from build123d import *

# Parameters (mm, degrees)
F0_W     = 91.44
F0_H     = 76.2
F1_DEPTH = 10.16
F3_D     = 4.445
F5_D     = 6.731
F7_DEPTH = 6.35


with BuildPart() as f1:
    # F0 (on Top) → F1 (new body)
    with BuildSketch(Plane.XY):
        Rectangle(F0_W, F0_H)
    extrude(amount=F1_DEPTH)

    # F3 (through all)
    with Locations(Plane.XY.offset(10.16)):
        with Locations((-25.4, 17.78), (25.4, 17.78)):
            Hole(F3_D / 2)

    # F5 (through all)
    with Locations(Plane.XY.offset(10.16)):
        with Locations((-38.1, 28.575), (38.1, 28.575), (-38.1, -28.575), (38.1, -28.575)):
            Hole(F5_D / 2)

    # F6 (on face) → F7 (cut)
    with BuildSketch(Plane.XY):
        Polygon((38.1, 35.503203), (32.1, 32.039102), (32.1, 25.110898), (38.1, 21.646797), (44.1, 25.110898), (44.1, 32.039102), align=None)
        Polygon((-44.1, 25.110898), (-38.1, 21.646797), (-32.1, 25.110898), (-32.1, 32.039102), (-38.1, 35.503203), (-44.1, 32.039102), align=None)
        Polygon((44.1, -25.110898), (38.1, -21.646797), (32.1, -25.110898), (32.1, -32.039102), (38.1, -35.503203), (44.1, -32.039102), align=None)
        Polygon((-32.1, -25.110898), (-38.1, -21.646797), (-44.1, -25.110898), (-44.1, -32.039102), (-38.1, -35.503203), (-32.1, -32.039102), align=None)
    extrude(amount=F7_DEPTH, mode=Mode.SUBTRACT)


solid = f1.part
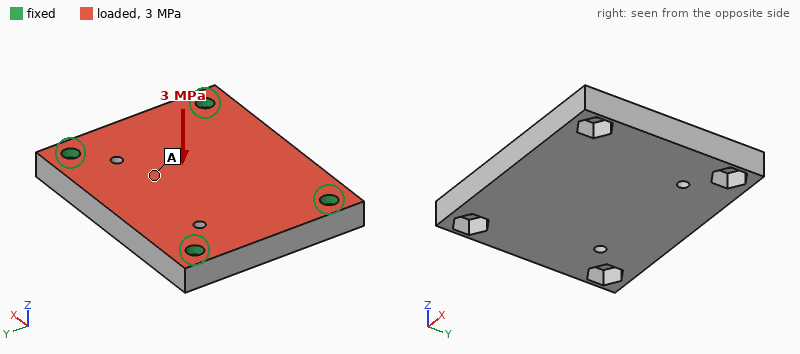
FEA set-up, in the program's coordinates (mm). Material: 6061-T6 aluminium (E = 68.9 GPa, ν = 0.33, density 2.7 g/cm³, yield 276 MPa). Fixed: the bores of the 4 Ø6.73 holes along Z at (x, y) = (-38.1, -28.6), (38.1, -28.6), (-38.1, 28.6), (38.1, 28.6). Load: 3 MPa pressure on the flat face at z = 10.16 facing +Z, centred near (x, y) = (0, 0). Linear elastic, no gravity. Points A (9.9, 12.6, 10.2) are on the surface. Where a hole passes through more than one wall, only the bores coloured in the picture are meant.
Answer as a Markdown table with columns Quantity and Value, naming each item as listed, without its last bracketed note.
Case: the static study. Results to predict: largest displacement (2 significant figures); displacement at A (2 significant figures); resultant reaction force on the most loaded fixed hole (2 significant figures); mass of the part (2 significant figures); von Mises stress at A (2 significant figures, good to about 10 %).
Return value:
| Quantity | Value |
|---|---|
| largest displacement | 0.12 mm |
| displacement at A | 0.11 mm |
| resultant reaction force on the most loaded fixed hole | 6.8 kN |
| mass of the part | 180 g |
| von Mises stress at A | 41 MPa |
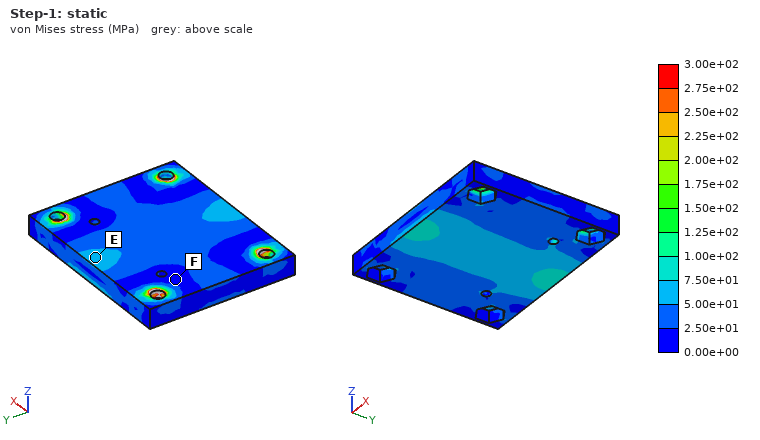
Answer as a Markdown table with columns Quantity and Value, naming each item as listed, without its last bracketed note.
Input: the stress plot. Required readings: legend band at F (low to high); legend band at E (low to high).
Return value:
| Quantity | Value |
|---|---|
| legend band at F | 0.00e+00 to 2.50e+01 MPa |
| legend band at E | 5.00e+01 to 7.50e+01 MPa |
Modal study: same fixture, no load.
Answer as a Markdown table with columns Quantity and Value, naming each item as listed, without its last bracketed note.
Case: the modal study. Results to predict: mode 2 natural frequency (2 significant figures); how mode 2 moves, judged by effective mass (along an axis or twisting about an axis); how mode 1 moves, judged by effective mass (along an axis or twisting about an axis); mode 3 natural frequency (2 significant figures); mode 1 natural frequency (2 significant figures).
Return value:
| Quantity | Value |
|---|---|
| mode 2 natural frequency | 7800 Hz |
| how mode 2 moves, judged by effective mass | twisting about X |
| how mode 1 moves, judged by effective mass | along Z |
| mode 3 natural frequency | 10 kHz |
| mode 1 natural frequency | 5400 Hz |
